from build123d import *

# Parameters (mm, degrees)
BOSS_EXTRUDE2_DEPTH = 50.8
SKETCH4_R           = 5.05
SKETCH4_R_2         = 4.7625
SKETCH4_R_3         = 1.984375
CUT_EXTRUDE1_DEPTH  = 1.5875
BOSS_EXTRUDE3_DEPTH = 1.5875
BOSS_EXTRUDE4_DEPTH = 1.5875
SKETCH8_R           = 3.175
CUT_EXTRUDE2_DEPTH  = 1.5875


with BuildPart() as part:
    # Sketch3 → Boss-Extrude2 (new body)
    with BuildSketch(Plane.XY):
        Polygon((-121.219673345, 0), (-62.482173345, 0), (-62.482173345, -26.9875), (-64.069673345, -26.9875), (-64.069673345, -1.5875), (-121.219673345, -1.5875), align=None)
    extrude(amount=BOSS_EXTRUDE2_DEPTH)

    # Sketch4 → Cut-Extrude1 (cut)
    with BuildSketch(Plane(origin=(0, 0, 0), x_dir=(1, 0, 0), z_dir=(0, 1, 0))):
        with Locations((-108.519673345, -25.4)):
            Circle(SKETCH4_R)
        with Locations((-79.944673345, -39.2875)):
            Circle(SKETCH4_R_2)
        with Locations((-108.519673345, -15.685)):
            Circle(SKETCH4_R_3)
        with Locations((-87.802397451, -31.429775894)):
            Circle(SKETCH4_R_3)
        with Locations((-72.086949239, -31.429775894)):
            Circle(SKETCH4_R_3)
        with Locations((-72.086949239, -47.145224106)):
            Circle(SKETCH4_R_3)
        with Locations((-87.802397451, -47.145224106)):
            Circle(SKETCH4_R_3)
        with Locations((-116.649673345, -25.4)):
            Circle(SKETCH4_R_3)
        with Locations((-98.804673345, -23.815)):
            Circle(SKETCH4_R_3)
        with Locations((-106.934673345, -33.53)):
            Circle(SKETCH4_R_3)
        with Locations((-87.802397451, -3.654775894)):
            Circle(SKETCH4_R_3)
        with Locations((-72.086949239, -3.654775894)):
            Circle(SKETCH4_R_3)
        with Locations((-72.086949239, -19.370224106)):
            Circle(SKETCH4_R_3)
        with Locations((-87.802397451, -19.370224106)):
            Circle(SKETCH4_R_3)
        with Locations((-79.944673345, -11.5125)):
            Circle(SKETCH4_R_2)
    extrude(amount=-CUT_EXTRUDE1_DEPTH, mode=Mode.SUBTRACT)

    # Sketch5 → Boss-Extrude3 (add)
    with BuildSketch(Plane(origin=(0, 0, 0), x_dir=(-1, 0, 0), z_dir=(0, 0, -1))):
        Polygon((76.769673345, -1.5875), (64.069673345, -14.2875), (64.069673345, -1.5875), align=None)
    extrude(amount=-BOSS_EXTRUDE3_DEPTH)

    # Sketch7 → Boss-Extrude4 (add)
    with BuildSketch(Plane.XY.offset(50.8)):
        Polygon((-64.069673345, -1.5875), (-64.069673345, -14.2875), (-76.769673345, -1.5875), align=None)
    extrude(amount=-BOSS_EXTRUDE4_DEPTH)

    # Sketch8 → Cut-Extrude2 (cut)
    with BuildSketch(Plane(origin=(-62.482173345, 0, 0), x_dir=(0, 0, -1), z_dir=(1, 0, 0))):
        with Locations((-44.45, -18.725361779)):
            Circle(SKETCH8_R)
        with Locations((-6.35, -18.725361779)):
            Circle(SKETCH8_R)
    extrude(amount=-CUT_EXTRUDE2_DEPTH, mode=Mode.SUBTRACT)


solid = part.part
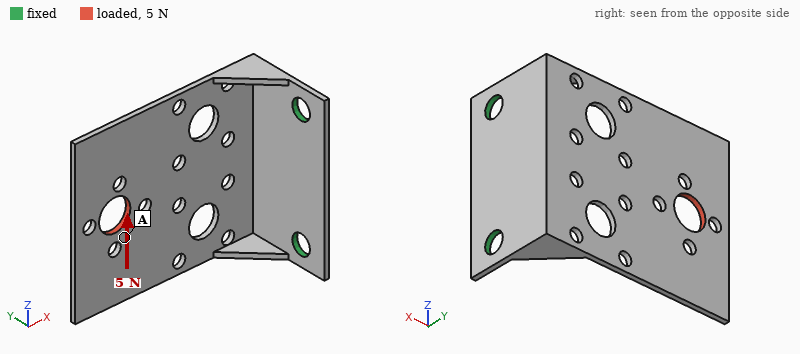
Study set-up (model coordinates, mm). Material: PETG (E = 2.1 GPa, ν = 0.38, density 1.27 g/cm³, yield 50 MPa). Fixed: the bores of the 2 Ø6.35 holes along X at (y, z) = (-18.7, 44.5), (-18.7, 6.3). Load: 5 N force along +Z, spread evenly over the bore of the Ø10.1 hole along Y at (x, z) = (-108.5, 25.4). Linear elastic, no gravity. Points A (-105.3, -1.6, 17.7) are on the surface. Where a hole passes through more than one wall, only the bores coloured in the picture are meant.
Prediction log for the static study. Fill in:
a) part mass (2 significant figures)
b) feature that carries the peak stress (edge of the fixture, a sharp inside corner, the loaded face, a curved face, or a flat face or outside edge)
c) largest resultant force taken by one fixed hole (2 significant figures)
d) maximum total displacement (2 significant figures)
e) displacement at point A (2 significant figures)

8.1 g
a flat face or outside edge
6.3 N
0.92 mm
0.55 mm
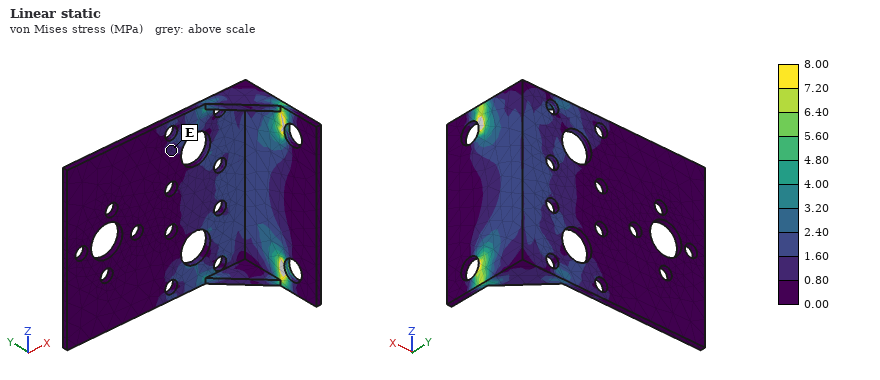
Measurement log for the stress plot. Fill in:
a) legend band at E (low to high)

0.80 to 1.60 MPa
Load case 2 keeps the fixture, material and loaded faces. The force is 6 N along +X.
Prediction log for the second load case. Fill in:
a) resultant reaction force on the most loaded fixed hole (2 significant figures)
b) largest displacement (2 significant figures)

3.0 N
0.93 mm
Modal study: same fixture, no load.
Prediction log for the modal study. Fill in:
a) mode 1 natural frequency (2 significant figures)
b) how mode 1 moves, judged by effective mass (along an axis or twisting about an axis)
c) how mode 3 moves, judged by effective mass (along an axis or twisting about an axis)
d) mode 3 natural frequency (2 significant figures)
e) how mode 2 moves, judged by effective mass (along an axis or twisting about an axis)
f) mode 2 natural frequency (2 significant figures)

86 Hz
along Y
along Z
350 Hz
along Z
210 Hz
